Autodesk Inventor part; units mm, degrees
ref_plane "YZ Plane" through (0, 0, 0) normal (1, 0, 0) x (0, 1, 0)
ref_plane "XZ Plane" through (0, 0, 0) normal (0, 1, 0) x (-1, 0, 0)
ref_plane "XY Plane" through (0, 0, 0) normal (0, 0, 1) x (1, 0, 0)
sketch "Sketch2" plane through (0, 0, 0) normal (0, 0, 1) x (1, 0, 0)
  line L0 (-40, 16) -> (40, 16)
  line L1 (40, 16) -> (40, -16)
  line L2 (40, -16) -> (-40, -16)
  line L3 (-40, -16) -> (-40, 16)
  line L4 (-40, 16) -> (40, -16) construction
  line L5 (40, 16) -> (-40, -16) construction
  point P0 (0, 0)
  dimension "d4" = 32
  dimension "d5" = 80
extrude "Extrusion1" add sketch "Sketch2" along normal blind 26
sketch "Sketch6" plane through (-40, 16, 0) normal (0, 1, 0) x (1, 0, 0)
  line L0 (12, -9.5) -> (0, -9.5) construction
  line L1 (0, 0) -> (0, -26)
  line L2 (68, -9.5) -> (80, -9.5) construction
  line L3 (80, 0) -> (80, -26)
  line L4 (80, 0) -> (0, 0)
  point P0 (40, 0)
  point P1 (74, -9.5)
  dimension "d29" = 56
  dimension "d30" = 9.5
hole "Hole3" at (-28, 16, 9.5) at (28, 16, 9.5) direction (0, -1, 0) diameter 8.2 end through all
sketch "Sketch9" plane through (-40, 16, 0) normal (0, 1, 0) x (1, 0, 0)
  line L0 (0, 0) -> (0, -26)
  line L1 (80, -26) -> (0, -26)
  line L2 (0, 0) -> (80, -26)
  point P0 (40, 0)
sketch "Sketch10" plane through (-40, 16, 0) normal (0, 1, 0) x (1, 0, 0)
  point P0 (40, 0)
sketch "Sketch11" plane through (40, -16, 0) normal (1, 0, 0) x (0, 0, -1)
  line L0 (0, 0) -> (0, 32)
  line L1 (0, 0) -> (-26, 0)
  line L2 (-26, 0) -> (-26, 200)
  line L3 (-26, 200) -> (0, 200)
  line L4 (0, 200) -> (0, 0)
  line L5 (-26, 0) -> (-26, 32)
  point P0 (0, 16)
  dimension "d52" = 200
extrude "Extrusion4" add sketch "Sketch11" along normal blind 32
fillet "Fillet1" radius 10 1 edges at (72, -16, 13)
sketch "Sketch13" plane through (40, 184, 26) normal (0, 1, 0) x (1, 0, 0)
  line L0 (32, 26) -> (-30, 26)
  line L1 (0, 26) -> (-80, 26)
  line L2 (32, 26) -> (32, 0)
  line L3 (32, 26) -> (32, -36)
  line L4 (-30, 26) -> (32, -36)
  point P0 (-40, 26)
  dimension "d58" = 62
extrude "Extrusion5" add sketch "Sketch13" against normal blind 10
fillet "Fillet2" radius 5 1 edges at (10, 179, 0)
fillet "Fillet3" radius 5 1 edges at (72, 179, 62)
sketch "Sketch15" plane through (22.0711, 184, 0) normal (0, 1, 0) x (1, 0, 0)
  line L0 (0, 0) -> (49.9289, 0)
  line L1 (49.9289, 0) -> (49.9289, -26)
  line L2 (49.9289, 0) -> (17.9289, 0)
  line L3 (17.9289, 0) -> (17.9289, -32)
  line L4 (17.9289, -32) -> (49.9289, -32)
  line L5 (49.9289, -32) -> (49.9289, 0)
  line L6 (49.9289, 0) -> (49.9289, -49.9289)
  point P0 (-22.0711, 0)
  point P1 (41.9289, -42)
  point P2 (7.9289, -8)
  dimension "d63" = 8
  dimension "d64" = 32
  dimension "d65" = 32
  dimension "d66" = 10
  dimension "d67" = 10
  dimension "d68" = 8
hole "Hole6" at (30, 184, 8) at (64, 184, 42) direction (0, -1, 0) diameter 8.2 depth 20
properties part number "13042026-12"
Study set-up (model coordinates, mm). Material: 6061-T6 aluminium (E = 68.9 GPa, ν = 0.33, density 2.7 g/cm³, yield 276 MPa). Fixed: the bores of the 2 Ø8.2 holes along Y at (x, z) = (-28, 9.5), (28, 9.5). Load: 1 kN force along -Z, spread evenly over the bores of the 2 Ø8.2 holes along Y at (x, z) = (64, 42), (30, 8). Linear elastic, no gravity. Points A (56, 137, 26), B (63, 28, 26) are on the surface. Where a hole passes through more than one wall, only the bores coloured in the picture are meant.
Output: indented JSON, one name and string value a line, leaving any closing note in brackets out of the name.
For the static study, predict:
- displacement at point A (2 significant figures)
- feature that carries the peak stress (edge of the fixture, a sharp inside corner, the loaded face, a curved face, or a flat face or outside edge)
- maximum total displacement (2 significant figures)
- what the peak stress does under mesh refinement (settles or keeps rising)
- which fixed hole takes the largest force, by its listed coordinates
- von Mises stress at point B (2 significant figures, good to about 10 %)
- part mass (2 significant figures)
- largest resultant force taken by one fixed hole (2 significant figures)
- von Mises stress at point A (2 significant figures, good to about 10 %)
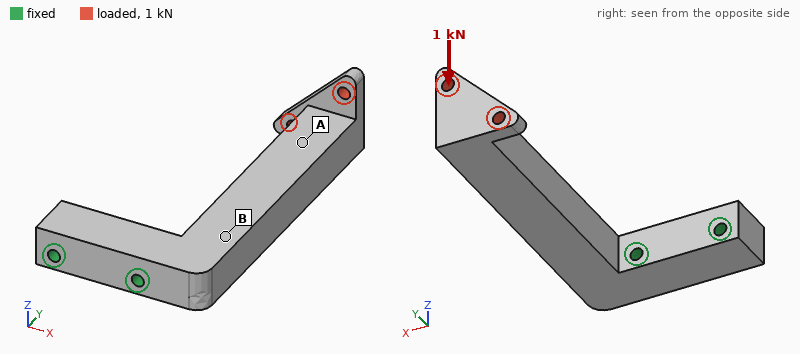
{
  "displacement at point A": "0.55 mm",
  "feature that carries the peak stress": "edge of the fixture",
  "maximum total displacement": "0.86 mm",
  "what the peak stress does under mesh refinement": "keeps rising",
  "which fixed hole takes the largest force, by its listed coordinates": "(28, 9.5)",
  "von Mises stress at point B": "39 MPa",
  "part mass": "640 g",
  "largest resultant force taken by one fixed hole": "1.2 kN",
  "von Mises stress at point A": "12 MPa"
}
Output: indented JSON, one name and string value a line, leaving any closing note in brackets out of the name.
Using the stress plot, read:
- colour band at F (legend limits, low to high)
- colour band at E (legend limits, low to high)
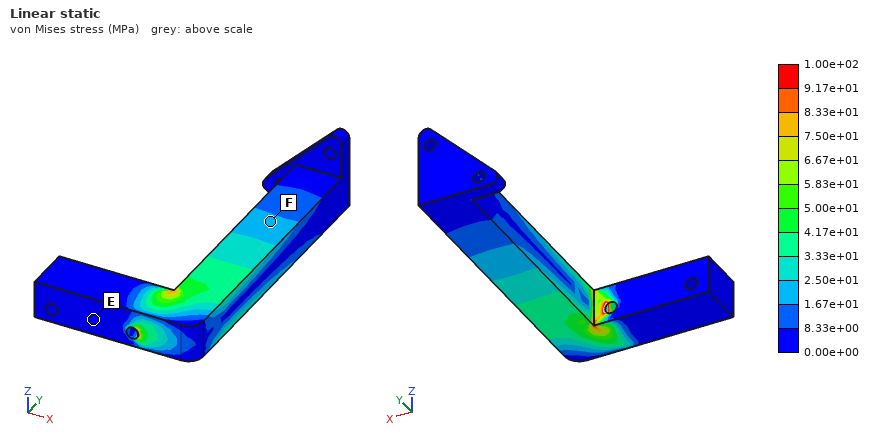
{
  "colour band at F": "1.67e+01 to 2.50e+01 MPa",
  "colour band at E": "0.00e+00 to 8.33e+00 MPa"
}
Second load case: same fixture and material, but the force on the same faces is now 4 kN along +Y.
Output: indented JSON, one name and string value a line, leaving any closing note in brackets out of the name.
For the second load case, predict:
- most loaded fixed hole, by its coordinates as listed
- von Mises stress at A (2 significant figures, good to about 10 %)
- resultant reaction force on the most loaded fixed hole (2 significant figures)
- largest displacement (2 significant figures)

{
  "most loaded fixed hole, by its coordinates as listed": "(28, 9.5)",
  "von Mises stress at A": "18 MPa",
  "resultant reaction force on the most loaded fixed hole": "4.1 kN",
  "largest displacement": "0.40 mm"
}
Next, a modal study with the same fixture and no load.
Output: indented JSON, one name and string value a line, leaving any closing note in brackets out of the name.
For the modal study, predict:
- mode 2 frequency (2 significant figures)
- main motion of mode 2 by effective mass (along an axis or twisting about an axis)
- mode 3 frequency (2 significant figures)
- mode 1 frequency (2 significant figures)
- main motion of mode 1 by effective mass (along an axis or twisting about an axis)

{
  "mode 2 frequency": "580 Hz",
  "main motion of mode 2 by effective mass": "along X",
  "mode 3 frequency": "2500 Hz",
  "mode 1 frequency": "470 Hz",
  "main motion of mode 1 by effective mass": "along Z"
}
